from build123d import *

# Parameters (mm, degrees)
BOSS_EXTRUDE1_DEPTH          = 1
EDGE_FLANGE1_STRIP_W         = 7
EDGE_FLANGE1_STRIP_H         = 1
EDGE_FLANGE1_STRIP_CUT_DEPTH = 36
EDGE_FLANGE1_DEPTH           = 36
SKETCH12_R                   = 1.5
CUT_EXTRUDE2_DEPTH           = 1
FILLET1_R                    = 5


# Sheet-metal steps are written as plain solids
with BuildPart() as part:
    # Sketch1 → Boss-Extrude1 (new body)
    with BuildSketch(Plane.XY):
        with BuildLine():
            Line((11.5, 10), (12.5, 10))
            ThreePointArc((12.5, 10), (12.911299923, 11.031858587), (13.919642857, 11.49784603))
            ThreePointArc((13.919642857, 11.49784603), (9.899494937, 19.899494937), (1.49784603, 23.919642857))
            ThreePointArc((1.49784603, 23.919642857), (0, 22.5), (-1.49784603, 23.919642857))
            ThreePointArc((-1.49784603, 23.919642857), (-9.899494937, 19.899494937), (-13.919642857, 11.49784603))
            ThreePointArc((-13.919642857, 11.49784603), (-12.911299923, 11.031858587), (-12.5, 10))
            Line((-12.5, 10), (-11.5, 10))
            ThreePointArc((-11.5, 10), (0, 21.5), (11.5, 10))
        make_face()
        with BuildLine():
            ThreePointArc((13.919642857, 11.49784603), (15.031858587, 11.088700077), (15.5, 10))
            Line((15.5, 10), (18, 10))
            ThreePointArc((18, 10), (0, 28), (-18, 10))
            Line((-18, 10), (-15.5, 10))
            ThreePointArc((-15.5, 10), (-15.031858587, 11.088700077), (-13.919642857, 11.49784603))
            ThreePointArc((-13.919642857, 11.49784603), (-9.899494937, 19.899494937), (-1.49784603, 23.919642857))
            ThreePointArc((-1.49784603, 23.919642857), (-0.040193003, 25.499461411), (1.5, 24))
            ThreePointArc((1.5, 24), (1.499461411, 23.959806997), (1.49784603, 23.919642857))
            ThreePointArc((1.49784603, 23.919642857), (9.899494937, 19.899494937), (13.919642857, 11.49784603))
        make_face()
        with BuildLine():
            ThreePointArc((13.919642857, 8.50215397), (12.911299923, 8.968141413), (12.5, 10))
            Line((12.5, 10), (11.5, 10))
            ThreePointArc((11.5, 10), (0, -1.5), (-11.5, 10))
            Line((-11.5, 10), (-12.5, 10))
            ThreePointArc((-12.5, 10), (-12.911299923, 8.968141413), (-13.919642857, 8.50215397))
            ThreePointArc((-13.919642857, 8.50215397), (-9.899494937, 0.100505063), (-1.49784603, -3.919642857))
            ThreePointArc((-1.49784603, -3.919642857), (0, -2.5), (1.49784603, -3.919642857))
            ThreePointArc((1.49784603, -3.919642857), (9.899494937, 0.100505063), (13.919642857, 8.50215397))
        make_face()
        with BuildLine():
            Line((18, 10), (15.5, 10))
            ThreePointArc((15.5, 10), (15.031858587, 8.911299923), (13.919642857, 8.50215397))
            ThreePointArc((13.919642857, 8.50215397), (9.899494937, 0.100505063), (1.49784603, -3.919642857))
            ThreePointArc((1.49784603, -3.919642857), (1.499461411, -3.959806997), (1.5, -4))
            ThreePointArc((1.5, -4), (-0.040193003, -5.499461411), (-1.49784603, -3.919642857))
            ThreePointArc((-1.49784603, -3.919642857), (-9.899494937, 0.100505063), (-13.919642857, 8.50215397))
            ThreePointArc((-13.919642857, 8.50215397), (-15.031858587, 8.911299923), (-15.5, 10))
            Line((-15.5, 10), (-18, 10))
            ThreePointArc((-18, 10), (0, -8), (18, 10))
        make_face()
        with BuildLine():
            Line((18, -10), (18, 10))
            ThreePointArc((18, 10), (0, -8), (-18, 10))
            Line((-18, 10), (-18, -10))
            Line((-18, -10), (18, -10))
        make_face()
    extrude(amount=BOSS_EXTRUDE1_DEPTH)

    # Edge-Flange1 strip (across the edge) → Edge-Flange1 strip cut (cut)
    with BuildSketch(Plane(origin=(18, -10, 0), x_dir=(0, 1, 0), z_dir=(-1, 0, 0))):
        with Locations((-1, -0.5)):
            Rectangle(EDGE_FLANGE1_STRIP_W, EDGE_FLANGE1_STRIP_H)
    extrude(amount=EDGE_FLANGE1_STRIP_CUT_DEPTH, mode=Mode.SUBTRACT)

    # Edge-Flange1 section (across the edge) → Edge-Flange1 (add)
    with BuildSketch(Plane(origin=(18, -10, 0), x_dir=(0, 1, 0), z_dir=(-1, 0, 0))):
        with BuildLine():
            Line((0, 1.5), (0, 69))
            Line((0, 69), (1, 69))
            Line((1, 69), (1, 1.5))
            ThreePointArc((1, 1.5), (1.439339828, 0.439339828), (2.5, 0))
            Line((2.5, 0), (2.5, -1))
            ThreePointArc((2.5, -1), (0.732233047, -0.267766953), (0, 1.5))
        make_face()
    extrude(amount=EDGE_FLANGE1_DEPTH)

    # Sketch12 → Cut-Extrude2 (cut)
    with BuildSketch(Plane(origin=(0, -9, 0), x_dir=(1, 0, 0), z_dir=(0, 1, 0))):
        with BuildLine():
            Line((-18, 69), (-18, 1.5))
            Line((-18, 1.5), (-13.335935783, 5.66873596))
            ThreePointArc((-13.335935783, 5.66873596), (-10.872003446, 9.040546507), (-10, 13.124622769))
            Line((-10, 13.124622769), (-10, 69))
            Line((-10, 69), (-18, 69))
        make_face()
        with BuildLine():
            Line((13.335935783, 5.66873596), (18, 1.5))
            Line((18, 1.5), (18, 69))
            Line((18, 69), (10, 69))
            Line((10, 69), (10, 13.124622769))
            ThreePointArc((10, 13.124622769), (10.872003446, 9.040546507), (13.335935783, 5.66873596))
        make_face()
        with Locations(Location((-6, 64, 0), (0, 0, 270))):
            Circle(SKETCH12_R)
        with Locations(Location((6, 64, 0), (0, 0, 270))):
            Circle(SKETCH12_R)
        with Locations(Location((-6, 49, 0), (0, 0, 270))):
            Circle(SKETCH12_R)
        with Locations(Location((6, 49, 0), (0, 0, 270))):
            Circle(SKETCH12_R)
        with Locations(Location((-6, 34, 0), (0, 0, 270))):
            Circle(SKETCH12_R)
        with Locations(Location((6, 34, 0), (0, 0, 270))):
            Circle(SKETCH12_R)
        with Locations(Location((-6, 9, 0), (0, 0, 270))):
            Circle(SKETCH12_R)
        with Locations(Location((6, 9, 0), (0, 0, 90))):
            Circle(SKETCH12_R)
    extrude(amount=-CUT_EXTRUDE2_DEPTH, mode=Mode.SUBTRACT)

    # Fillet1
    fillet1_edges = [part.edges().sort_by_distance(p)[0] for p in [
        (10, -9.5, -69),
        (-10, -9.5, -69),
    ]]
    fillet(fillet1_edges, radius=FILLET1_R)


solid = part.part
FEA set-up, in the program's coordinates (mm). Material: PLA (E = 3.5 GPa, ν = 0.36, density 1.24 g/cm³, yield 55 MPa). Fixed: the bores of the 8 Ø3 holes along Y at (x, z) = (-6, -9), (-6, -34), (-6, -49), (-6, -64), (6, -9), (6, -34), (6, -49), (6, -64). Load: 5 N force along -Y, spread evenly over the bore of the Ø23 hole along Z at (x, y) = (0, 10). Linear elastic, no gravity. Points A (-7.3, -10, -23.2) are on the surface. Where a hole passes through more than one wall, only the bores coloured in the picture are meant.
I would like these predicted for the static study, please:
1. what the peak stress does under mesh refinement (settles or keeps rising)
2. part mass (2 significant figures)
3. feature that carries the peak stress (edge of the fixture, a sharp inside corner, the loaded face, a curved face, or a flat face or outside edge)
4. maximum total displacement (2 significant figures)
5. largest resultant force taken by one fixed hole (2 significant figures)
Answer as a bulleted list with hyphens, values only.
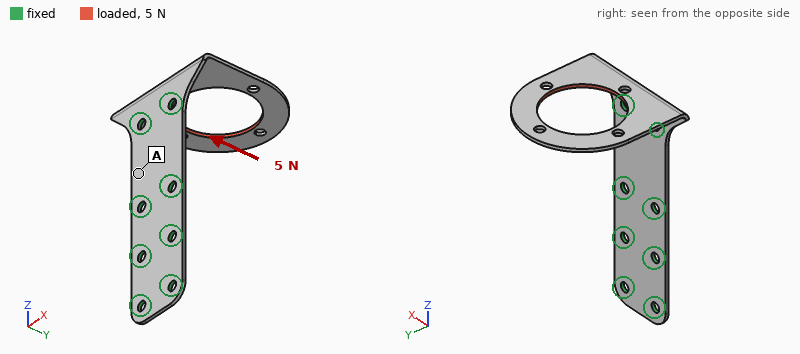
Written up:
- keeps rising
- 2.7 g
- edge of the fixture
- 0.90 mm
- 2.5 N
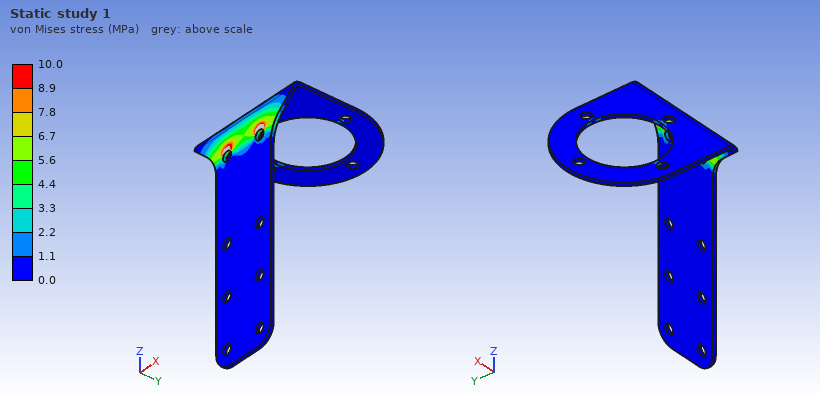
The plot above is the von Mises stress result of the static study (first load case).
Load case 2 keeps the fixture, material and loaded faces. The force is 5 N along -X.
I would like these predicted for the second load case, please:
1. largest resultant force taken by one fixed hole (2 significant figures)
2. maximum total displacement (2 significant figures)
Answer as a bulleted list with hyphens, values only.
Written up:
- 7.5 N
- 0.93 mm
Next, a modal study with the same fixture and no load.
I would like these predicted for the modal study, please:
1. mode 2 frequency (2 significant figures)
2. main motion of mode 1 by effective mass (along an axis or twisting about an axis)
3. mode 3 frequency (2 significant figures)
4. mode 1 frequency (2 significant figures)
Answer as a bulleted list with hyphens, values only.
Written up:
- 390 Hz
- along Z
- 580 Hz
- 170 Hz
